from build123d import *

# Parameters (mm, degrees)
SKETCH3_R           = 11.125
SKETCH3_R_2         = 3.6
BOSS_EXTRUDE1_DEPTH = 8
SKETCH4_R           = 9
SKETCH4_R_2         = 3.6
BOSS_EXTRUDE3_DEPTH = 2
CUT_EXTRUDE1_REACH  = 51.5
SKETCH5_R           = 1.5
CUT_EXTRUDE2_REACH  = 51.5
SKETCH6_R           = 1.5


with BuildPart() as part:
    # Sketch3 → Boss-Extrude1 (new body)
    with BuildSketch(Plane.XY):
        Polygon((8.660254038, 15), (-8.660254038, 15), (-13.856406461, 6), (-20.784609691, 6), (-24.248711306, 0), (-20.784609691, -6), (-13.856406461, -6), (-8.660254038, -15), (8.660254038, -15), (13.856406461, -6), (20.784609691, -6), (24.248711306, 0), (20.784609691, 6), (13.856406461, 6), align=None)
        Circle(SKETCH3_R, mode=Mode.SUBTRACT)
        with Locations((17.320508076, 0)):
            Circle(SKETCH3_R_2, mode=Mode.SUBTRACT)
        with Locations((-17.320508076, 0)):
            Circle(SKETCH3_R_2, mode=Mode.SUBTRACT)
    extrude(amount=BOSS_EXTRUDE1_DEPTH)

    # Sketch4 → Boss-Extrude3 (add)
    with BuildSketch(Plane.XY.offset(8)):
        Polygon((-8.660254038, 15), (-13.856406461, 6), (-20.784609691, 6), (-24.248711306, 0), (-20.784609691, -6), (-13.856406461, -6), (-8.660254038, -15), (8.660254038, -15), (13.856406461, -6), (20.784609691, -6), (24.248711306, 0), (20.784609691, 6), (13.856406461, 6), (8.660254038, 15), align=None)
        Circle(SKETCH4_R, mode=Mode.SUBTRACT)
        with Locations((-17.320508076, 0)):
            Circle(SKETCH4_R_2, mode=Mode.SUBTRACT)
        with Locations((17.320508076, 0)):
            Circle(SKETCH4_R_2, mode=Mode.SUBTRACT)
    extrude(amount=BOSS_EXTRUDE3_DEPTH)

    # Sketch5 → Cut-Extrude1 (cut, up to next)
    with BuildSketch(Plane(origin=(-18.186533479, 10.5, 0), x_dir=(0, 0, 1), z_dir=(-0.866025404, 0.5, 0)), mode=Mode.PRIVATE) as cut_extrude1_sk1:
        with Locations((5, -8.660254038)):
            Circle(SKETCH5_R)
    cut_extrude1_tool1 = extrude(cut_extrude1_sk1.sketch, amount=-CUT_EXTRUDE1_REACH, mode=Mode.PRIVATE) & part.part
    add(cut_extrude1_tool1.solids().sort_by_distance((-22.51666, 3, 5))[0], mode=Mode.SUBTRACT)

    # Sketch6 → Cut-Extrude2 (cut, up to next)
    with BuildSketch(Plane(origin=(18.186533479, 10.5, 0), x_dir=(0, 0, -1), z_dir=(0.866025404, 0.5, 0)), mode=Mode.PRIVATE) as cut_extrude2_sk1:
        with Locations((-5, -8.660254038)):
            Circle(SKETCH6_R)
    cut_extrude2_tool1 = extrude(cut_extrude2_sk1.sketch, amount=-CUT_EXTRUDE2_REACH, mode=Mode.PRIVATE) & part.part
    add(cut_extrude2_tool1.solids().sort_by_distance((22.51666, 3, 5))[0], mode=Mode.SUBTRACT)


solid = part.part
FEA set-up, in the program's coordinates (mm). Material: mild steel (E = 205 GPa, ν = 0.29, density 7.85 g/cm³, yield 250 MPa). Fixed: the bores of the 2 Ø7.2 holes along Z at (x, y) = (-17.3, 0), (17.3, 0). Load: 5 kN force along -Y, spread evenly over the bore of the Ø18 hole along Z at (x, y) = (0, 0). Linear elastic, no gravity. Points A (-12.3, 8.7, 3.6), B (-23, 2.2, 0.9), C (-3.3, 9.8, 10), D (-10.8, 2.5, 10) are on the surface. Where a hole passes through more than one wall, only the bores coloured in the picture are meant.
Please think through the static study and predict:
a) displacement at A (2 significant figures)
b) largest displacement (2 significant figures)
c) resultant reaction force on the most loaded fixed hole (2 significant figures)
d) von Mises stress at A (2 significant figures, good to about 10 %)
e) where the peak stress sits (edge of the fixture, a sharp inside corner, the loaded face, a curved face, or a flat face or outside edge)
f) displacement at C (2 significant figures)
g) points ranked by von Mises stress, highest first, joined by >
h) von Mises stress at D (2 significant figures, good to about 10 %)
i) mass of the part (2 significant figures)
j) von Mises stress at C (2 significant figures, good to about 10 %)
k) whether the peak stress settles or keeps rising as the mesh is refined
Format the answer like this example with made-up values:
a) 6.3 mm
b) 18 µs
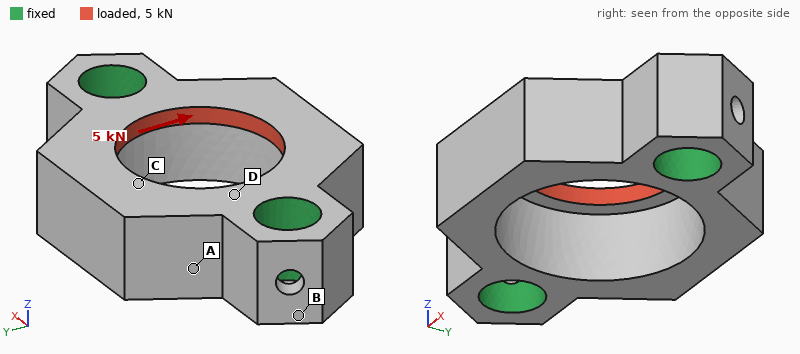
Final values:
a) 1.9 µm
b) 9.6 µm
c) 2.5 kN
d) 29 MPa
e) edge of the fixture
f) 7.6 µm
g) D > C > A > B
h) 83 MPa
i) 39 g
j) 65 MPa
k) keeps rising
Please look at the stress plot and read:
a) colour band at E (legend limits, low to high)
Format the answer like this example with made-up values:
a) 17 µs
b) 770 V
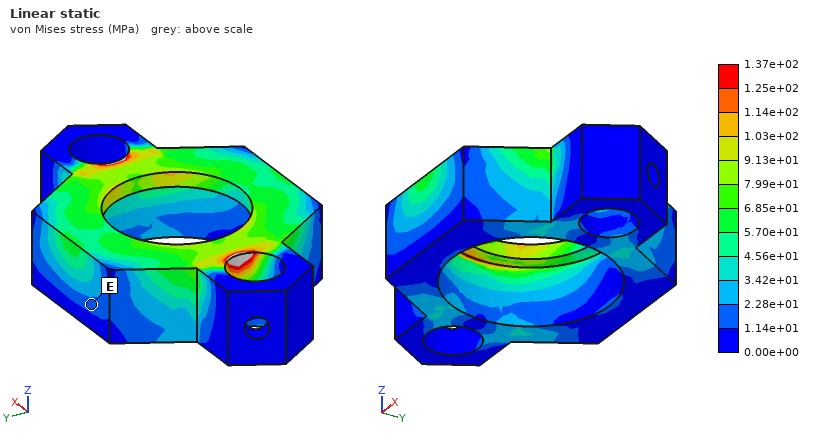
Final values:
a) 1.14e+01 to 2.28e+01 MPa
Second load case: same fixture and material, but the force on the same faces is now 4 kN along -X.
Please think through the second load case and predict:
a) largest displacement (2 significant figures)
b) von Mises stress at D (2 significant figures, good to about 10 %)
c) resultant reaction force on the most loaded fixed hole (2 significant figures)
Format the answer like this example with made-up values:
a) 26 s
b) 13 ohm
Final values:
a) 4.4 µm
b) 63 MPa
c) 2.0 kN
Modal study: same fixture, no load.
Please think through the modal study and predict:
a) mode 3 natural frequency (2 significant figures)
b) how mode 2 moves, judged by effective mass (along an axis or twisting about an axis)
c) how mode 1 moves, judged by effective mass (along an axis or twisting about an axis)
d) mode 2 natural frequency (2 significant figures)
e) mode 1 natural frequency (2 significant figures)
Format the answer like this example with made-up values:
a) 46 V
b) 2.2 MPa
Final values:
a) 33 kHz
b) along Z
c) twisting about X
d) 22 kHz
e) 21 kHz
